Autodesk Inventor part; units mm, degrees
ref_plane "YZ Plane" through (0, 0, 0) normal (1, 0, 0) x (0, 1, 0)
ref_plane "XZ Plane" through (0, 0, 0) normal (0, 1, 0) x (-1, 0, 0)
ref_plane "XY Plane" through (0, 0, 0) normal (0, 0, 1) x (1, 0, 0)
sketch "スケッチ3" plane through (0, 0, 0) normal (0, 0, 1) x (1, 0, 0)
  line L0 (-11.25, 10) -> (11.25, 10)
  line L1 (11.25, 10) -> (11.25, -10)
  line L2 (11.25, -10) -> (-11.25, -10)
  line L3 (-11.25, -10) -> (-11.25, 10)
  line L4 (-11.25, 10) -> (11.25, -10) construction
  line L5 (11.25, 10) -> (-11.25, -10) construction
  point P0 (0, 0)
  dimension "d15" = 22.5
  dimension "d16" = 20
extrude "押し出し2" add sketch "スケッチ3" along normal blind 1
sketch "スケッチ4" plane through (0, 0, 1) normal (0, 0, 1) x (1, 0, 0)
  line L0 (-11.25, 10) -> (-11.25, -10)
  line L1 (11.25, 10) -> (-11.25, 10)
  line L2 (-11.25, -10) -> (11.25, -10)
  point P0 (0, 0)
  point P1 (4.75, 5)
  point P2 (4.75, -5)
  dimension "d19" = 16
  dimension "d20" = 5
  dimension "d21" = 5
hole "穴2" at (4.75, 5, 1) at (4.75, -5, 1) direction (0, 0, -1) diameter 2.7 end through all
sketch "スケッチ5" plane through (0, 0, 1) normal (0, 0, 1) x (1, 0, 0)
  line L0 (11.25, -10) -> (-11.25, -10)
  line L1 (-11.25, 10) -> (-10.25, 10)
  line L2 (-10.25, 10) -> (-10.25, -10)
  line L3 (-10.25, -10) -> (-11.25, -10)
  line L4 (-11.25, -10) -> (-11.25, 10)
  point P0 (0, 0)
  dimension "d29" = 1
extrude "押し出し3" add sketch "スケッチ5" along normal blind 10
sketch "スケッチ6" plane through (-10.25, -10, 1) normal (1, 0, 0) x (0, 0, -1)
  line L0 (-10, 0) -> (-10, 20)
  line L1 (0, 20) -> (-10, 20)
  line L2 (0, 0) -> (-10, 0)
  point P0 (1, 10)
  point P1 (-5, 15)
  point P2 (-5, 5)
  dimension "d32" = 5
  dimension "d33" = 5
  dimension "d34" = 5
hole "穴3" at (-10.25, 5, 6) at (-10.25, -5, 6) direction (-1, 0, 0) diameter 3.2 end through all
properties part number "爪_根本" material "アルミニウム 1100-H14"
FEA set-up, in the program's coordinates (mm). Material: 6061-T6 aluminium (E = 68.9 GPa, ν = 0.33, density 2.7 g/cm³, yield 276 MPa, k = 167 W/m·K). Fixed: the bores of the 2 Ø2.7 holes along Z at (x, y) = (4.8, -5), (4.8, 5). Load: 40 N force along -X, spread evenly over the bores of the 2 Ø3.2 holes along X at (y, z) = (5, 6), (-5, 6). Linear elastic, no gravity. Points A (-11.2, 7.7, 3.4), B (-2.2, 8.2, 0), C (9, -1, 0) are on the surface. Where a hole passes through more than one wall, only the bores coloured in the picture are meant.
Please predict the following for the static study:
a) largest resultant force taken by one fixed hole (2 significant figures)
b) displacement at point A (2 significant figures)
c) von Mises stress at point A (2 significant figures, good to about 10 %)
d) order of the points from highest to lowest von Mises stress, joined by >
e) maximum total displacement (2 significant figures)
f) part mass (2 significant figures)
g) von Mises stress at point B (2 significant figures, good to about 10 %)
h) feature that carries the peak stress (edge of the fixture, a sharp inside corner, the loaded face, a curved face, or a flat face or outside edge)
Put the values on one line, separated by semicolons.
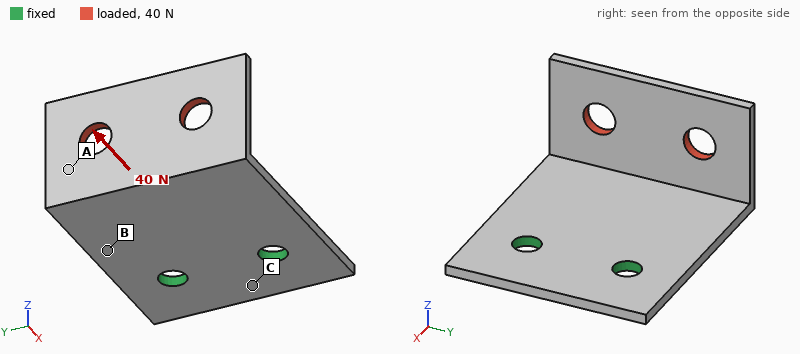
20 N; 0.23 mm; 29 MPa; B > A > C; 0.38 mm; 1.7 g; 63 MPa; a flat face or outside edge
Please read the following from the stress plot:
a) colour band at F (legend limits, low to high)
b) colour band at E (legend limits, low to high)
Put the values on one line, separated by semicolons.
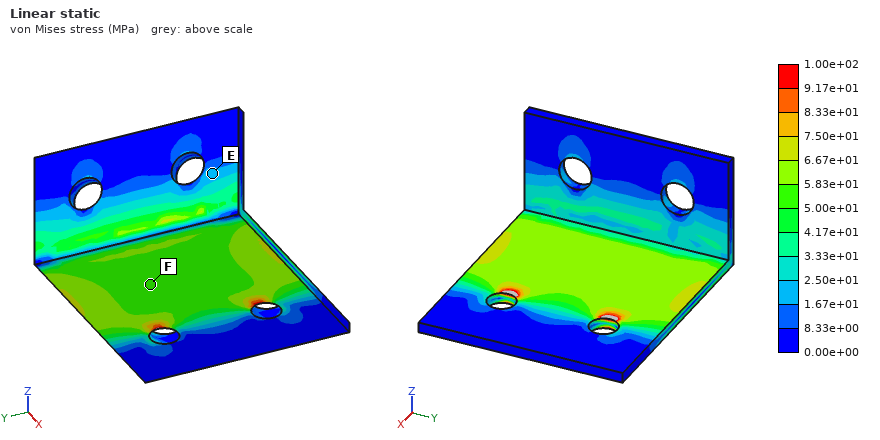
5.00e+01 to 5.83e+01 MPa; 1.67e+01 to 2.50e+01 MPa
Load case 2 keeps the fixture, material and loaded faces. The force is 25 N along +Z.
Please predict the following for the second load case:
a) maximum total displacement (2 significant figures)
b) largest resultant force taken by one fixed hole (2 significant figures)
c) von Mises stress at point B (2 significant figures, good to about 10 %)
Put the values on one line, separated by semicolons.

0.33 mm; 13 N; 63 MPa
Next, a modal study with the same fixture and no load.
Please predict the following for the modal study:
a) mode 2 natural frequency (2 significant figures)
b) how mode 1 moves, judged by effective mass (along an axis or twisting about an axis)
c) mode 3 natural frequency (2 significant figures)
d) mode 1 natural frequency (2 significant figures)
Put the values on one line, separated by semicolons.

3300 Hz; along Z; 5500 Hz; 1700 Hz
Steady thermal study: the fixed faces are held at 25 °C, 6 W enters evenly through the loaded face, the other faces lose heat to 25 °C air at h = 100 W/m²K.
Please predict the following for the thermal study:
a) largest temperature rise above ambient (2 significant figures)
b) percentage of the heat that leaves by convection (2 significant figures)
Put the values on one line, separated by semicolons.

31 K; 30 %
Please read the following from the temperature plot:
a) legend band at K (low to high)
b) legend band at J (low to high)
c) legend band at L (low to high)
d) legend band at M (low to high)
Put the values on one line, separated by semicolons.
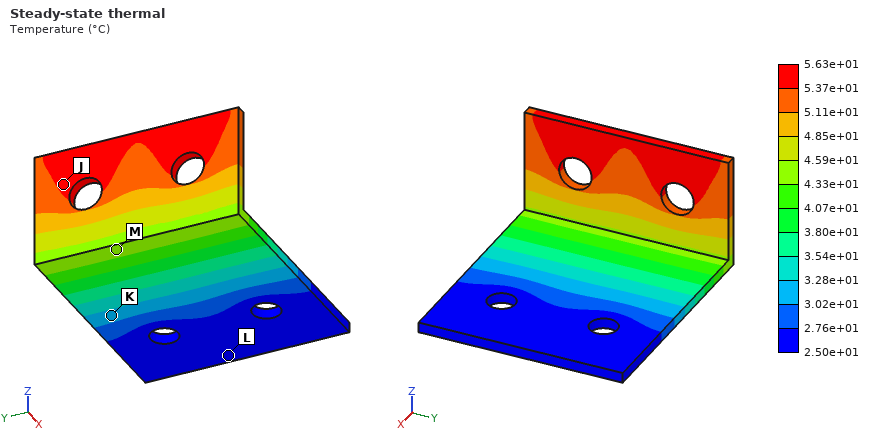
3.02e+01 to 3.28e+01 °C; 5.37e+01 to 5.63e+01 °C; 2.50e+01 to 2.76e+01 °C; 4.33e+01 to 4.59e+01 °C
